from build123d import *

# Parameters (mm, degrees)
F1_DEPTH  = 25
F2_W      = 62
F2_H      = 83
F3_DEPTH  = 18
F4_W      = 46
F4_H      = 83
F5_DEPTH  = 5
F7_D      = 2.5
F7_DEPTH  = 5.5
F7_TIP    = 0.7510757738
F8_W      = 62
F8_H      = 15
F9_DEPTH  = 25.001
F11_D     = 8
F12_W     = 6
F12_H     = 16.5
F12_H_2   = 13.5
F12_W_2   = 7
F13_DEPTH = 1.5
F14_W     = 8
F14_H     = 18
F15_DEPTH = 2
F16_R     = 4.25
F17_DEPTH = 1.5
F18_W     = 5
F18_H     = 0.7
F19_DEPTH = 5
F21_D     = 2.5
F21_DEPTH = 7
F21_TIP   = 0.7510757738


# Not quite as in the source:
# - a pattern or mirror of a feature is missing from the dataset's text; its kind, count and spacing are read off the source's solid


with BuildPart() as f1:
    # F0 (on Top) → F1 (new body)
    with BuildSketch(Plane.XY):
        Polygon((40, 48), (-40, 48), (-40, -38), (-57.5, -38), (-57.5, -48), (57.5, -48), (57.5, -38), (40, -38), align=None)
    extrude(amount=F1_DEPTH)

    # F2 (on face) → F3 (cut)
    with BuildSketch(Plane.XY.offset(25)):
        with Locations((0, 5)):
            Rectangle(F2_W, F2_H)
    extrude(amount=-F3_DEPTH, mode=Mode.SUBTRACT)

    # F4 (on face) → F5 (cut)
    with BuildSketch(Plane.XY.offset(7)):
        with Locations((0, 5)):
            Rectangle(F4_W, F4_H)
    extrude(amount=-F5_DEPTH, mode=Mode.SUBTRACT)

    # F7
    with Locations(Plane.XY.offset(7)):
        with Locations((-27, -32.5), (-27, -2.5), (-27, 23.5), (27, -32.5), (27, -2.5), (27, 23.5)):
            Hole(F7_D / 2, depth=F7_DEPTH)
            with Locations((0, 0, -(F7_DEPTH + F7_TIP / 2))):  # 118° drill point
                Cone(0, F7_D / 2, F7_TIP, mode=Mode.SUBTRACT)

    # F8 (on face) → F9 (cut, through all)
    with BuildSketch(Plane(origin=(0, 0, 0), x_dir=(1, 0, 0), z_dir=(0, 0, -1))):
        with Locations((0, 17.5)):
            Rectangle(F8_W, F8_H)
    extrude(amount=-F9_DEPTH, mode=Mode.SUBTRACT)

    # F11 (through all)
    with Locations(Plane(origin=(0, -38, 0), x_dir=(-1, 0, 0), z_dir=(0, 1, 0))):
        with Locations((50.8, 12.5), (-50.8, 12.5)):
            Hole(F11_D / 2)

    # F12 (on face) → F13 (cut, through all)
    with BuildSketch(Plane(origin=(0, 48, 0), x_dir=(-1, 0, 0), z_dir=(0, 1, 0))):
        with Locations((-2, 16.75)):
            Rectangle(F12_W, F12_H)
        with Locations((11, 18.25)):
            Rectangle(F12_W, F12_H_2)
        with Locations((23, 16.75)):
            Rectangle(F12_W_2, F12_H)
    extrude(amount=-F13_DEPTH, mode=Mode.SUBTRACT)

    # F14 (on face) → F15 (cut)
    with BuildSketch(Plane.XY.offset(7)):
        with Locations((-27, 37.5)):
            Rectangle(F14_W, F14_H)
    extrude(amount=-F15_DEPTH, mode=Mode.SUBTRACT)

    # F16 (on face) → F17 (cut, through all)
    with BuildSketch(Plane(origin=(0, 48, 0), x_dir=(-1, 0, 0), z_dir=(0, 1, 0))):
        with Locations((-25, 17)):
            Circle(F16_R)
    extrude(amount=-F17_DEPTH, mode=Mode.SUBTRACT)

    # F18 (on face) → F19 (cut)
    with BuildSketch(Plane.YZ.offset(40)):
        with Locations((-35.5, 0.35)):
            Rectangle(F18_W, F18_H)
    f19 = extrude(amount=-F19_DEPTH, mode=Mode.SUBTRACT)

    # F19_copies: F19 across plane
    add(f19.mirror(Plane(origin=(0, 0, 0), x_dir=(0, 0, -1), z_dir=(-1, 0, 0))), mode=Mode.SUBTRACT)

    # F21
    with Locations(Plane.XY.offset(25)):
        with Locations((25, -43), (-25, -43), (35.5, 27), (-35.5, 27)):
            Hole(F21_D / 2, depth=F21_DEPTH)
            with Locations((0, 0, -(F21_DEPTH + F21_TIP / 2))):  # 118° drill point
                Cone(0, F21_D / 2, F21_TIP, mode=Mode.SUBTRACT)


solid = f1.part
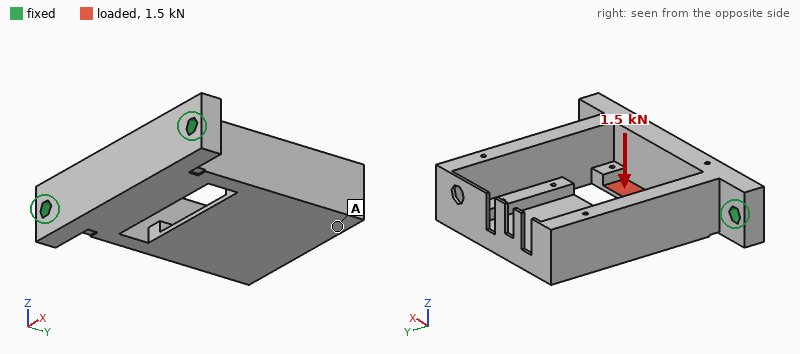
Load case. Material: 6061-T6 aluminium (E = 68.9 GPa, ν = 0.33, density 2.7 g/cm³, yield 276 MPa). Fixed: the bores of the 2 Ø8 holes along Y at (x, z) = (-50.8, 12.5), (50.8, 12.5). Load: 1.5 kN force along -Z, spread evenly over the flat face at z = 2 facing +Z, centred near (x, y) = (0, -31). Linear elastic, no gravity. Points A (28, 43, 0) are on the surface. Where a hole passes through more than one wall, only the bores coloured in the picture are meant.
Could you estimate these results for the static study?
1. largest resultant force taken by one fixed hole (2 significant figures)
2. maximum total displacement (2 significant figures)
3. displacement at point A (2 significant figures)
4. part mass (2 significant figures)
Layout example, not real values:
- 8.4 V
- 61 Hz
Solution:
- 760 N
- 0.16 mm
- 0.056 mm
- 230 g
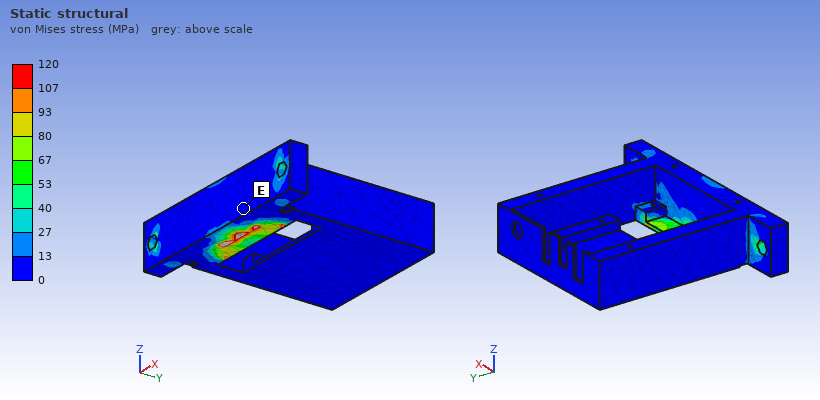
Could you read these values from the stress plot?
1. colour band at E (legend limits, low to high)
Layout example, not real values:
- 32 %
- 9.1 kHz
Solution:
- 0 to 13 MPa
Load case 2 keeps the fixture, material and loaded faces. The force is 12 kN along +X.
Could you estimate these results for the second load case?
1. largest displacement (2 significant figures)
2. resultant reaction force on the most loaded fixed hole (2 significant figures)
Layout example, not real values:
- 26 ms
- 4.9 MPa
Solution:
- 58 µm
- 6.4 kN
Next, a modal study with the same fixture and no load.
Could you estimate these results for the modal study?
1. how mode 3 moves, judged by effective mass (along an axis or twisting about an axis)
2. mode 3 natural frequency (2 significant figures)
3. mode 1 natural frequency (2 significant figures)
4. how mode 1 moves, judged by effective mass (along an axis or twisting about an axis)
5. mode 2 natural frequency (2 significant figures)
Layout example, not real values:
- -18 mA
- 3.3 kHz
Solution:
- along X
- 2800 Hz
- 1100 Hz
- along Z
- 1600 Hz
